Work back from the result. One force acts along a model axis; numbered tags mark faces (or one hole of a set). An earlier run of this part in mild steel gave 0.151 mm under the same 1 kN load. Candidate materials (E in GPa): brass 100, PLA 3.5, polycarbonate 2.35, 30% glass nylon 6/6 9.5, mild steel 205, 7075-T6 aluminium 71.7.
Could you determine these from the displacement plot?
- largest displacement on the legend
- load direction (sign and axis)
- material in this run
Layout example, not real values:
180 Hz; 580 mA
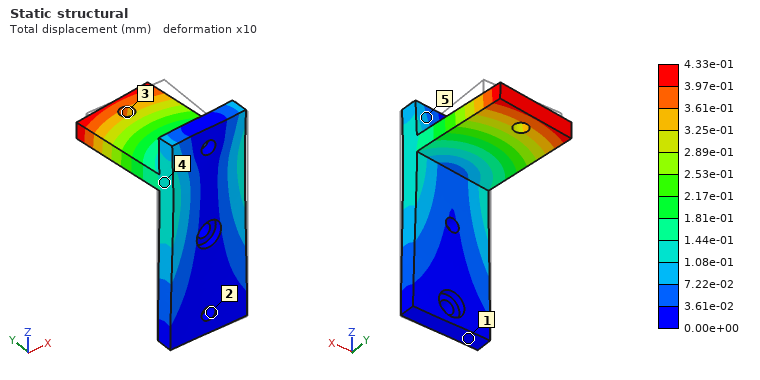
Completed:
4.33e-01 mm; -X; 7075-T6 aluminium
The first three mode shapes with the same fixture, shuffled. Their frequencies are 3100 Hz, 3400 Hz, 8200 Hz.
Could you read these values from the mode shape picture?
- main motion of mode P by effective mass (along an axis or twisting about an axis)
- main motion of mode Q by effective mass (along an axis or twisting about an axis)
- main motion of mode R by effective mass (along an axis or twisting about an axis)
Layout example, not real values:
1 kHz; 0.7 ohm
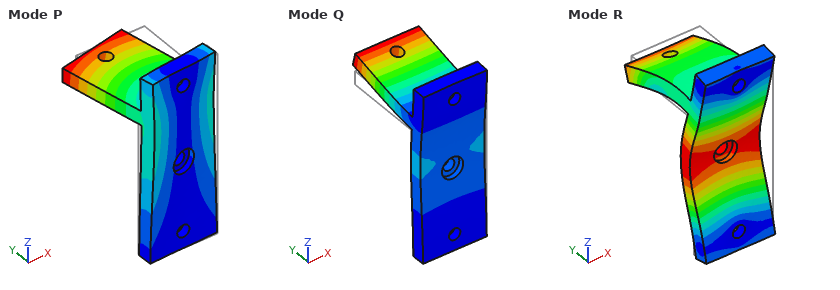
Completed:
along X; along Z; along Y
